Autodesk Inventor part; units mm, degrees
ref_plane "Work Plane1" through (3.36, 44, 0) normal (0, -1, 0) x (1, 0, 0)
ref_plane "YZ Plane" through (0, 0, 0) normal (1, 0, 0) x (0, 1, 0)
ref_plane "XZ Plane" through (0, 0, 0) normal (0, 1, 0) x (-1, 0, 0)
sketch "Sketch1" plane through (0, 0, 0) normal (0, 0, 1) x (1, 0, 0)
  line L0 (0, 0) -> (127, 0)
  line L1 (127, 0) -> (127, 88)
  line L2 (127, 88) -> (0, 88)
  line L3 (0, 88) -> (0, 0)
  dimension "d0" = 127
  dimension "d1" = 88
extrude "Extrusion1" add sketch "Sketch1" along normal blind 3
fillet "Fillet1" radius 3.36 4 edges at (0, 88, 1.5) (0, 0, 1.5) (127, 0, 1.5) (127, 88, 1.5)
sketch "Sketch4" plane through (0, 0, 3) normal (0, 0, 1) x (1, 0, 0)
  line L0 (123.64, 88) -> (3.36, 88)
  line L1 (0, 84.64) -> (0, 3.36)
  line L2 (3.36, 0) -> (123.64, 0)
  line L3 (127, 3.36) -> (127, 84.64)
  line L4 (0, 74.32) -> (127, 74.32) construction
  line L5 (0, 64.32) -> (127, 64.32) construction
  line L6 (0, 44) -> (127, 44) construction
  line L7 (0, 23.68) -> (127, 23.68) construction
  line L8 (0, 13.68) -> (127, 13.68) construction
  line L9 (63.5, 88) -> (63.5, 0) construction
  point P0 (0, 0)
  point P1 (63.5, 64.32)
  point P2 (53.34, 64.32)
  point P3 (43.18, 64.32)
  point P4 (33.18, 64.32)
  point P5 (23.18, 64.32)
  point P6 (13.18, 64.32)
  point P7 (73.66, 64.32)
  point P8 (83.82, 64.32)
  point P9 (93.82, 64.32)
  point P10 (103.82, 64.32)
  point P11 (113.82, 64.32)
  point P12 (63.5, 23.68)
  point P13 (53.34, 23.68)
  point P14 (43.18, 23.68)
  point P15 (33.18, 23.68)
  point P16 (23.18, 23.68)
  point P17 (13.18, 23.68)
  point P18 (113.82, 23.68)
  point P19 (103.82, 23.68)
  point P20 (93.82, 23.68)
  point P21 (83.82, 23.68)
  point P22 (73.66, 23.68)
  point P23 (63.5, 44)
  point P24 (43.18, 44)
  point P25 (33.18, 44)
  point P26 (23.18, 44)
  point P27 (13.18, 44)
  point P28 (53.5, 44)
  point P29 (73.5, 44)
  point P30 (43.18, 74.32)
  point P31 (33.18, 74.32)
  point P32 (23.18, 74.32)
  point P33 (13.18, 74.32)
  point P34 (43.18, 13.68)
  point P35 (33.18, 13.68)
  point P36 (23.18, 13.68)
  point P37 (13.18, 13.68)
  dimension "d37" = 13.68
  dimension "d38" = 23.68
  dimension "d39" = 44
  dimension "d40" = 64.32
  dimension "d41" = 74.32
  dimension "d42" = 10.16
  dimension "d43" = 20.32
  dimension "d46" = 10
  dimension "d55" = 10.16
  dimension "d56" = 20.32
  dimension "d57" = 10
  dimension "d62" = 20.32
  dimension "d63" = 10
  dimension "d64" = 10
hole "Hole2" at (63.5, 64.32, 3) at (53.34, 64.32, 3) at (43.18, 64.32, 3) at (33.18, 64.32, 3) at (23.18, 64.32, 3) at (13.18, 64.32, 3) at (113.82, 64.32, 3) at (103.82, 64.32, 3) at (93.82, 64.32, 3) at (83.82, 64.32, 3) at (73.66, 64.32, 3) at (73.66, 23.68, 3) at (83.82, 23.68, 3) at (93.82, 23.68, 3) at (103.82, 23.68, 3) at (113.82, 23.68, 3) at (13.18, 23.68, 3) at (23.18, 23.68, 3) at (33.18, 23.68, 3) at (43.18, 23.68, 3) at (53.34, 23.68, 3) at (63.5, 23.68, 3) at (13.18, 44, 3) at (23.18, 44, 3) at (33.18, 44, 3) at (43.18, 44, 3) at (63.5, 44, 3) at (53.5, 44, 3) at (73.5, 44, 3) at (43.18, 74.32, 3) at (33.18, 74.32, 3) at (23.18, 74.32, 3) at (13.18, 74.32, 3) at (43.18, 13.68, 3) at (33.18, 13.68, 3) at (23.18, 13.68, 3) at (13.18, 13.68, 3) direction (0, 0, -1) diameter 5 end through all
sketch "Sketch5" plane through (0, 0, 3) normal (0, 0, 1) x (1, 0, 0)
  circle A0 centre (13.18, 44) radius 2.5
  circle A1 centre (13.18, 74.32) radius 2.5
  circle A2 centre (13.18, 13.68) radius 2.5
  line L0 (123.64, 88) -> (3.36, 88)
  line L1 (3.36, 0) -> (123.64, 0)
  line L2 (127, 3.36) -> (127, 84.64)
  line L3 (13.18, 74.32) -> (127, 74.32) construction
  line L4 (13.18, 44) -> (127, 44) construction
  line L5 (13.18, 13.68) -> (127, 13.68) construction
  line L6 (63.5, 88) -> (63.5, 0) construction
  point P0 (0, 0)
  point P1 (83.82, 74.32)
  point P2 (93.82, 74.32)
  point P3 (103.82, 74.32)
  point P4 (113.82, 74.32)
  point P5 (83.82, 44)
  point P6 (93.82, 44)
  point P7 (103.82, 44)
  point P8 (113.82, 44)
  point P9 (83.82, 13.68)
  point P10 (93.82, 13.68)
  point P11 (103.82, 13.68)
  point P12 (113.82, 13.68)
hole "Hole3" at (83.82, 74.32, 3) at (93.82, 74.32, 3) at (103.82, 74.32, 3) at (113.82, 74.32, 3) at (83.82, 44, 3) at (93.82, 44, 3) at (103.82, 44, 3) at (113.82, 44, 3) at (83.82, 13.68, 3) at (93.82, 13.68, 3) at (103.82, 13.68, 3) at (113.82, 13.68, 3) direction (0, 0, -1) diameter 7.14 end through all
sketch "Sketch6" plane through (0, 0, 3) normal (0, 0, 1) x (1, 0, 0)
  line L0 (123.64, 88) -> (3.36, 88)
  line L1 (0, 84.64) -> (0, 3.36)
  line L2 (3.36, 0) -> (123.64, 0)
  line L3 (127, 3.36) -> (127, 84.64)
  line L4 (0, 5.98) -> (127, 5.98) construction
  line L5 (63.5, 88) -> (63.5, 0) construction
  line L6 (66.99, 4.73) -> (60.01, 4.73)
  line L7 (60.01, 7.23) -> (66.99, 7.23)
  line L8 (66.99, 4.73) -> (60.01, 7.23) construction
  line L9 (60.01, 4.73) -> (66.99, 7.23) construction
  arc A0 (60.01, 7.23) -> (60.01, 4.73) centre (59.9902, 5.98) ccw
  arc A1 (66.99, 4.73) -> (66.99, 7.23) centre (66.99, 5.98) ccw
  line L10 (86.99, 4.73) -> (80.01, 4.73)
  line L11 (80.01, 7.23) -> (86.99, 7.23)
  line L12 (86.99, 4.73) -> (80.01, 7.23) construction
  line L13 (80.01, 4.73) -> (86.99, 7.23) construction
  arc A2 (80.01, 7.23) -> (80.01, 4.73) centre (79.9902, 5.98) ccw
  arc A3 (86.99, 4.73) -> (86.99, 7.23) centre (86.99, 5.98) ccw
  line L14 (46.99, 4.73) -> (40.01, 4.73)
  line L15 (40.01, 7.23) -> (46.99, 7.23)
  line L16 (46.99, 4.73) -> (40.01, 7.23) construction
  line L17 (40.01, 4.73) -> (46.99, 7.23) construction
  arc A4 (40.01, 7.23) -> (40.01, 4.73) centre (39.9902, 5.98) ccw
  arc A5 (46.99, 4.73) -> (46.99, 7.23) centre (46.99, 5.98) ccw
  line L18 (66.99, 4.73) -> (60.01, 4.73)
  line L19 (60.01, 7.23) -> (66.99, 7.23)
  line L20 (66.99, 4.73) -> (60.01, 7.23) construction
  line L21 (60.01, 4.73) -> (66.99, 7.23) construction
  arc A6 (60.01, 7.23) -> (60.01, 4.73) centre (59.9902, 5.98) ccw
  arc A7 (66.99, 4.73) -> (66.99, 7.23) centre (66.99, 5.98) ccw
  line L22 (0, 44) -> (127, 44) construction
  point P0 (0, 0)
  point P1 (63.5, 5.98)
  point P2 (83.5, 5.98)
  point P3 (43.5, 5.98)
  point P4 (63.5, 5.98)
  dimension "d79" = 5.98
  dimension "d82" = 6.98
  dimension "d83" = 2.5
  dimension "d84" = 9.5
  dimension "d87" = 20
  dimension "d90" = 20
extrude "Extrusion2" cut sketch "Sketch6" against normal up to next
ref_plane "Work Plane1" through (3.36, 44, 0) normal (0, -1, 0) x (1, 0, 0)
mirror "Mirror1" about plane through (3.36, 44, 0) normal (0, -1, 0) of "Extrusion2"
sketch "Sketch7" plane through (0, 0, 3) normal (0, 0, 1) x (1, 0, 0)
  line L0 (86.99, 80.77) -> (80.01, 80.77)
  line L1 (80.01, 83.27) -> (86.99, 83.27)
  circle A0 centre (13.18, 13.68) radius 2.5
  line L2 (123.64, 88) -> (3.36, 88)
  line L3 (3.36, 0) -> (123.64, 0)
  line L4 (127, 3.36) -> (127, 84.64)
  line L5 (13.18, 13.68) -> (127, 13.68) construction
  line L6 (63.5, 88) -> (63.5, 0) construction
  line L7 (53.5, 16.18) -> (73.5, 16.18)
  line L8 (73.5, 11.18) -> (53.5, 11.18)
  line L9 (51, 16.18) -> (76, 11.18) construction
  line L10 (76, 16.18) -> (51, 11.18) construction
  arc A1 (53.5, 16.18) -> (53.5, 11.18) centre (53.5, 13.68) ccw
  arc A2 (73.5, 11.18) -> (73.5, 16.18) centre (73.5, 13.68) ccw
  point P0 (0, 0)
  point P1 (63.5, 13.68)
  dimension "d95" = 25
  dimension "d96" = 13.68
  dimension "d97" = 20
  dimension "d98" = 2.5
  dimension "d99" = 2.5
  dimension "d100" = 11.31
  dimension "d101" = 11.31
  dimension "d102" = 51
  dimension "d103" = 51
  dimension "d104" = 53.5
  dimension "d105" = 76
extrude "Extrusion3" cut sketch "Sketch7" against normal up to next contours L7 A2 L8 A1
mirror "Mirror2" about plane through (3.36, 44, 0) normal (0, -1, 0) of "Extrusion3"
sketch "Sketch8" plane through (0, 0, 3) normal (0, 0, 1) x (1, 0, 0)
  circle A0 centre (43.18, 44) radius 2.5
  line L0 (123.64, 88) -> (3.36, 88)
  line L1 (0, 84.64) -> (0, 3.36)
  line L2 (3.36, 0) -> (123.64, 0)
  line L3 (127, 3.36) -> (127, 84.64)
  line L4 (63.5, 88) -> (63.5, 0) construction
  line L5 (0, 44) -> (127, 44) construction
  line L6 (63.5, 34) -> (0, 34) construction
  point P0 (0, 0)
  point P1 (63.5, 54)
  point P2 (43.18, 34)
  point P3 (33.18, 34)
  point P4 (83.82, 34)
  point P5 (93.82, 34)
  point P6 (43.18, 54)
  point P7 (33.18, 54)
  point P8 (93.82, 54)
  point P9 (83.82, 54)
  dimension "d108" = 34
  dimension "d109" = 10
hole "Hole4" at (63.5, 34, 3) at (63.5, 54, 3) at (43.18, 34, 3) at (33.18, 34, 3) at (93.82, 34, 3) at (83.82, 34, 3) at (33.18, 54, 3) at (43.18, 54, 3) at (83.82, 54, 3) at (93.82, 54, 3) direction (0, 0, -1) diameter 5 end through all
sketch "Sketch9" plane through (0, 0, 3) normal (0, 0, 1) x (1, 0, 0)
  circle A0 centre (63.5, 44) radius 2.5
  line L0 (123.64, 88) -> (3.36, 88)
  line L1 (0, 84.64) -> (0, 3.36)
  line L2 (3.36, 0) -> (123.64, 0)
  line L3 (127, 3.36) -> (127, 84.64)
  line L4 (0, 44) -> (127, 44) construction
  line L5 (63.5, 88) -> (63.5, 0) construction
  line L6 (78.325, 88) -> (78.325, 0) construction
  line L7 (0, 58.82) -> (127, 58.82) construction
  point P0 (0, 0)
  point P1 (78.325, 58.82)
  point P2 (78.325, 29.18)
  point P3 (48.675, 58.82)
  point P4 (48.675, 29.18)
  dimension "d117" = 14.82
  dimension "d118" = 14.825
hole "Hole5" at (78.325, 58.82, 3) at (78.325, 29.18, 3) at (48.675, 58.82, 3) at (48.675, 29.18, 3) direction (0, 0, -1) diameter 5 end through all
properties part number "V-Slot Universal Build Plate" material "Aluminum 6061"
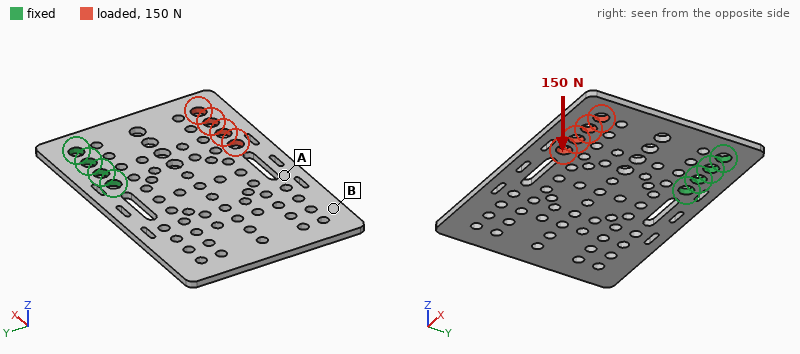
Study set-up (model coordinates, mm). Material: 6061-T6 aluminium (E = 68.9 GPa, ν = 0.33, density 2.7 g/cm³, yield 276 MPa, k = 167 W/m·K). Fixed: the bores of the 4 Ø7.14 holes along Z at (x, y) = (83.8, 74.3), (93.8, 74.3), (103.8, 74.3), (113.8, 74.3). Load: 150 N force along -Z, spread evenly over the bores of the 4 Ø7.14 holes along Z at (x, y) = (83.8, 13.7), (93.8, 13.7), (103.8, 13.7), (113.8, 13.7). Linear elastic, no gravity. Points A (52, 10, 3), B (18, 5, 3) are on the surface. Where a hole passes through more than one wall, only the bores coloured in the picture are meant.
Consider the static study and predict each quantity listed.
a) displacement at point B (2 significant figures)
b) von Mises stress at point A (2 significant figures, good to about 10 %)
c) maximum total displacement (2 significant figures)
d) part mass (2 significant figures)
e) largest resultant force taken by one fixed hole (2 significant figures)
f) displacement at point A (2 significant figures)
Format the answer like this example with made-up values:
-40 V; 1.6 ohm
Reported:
1.1 mm; 21 MPa; 1.6 mm; 75 g; 45 N; 1.1 mm
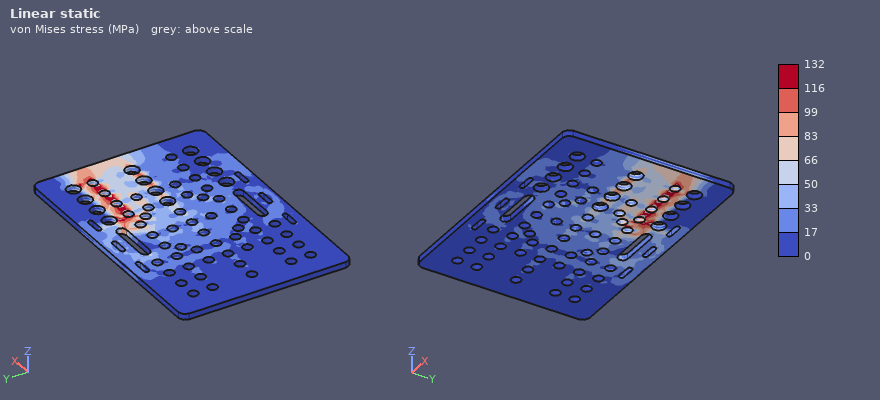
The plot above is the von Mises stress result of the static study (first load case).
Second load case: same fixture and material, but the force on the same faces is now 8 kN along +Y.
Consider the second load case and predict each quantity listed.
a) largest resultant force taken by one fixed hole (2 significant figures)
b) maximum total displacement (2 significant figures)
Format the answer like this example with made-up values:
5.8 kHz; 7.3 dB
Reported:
2.7 kN; 84 µm
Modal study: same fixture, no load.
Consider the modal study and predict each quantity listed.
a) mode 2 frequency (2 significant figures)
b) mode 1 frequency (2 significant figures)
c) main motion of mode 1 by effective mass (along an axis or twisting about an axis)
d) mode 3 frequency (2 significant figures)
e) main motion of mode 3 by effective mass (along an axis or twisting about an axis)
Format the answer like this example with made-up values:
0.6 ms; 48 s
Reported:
410 Hz; 220 Hz; along Z; 760 Hz; along Z
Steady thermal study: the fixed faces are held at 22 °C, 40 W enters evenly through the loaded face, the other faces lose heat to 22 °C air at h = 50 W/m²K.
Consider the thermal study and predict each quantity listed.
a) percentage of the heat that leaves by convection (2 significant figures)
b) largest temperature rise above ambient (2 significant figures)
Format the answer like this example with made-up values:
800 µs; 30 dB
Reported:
55 %; 67 K
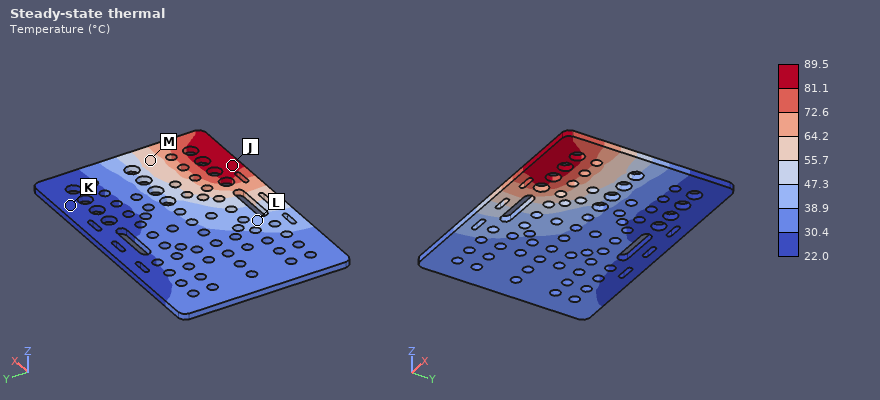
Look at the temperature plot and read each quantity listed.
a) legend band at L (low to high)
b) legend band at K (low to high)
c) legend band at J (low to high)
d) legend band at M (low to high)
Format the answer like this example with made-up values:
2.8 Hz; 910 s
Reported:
38.9 to 47.3 °C; 22.0 to 30.4 °C; 81.1 to 89.5 °C; 55.7 to 64.2 °C
